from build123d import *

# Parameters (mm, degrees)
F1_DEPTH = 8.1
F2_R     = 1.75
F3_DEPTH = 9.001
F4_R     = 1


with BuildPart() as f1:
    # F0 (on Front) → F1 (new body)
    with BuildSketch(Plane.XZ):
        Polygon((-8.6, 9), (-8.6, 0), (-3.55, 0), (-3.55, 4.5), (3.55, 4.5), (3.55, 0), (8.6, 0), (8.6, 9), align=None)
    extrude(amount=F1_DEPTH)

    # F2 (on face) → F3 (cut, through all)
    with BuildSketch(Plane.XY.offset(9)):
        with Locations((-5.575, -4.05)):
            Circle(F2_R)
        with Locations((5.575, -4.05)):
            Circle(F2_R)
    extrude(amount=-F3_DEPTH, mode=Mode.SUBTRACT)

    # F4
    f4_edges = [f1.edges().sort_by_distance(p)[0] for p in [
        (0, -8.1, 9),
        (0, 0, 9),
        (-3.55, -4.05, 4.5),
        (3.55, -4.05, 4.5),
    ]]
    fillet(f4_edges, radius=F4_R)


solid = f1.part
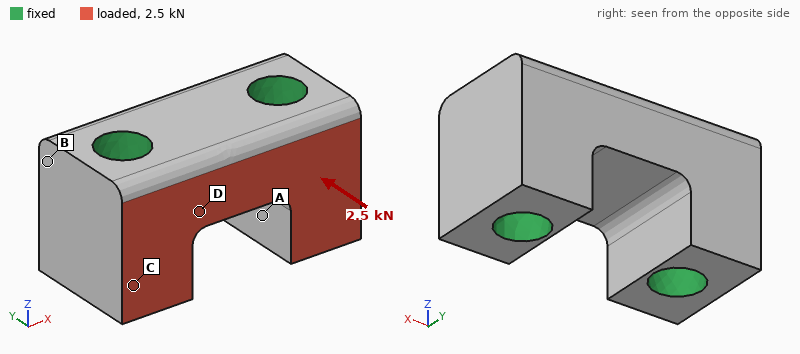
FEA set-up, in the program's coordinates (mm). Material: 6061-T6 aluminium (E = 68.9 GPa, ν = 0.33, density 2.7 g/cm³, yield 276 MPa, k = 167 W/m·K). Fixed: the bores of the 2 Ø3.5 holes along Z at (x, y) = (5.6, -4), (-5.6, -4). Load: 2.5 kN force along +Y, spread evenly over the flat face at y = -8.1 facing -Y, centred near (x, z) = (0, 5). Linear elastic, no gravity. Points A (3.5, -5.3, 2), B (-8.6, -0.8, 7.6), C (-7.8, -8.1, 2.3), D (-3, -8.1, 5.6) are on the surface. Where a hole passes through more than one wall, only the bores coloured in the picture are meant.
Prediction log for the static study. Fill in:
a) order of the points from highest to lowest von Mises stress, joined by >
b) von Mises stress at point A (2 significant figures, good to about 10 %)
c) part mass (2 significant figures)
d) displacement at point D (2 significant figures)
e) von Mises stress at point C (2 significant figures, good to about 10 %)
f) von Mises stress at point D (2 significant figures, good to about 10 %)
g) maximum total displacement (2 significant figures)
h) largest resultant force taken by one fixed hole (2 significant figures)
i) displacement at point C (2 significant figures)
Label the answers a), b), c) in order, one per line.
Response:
a) C > D > A > B
b) 12 MPa
c) 2.2 g
d) 1.4 µm
e) 24 MPa
f) 18 MPa
g) 2.3 µm
h) 1.3 kN
i) 1.4 µm
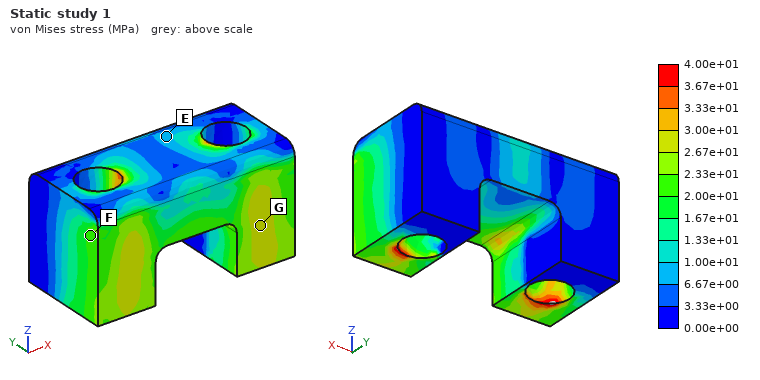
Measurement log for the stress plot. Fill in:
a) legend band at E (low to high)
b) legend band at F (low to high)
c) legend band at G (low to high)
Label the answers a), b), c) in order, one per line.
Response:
a) 6.67e+00 to 1.00e+01 MPa
b) 2.00e+01 to 2.33e+01 MPa
c) 2.67e+01 to 3.00e+01 MPa
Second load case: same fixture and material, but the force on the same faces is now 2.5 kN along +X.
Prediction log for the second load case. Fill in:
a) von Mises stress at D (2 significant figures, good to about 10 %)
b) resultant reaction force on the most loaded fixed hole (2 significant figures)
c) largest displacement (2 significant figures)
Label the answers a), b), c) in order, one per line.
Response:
a) 43 MPa
b) 1.3 kN
c) 6.0 µm
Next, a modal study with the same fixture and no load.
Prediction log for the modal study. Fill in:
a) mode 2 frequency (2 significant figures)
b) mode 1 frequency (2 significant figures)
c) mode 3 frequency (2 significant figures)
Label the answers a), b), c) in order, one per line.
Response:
a) 150 kHz
b) 150 kHz
c) 150 kHz
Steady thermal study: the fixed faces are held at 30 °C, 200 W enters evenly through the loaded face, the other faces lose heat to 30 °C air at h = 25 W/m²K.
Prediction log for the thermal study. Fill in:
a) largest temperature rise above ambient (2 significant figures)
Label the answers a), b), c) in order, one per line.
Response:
a) 41 K
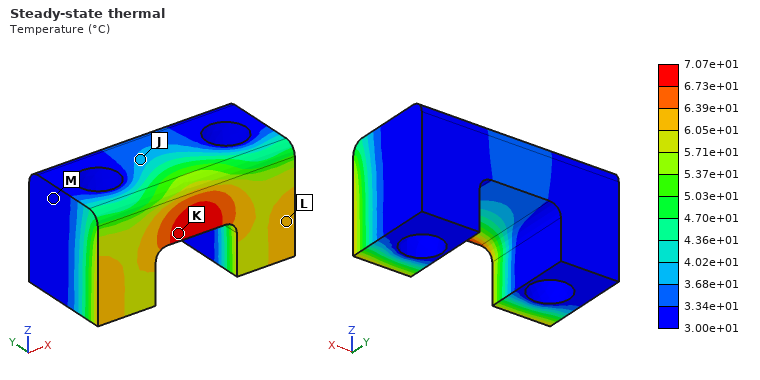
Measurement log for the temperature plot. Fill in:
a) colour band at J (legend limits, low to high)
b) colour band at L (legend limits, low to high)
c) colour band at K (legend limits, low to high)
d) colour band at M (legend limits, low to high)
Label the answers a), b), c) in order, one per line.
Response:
a) 3.68e+01 to 4.02e+01 °C
b) 6.05e+01 to 6.39e+01 °C
c) 6.73e+01 to 7.07e+01 °C
d) 3.00e+01 to 3.34e+01 °C
